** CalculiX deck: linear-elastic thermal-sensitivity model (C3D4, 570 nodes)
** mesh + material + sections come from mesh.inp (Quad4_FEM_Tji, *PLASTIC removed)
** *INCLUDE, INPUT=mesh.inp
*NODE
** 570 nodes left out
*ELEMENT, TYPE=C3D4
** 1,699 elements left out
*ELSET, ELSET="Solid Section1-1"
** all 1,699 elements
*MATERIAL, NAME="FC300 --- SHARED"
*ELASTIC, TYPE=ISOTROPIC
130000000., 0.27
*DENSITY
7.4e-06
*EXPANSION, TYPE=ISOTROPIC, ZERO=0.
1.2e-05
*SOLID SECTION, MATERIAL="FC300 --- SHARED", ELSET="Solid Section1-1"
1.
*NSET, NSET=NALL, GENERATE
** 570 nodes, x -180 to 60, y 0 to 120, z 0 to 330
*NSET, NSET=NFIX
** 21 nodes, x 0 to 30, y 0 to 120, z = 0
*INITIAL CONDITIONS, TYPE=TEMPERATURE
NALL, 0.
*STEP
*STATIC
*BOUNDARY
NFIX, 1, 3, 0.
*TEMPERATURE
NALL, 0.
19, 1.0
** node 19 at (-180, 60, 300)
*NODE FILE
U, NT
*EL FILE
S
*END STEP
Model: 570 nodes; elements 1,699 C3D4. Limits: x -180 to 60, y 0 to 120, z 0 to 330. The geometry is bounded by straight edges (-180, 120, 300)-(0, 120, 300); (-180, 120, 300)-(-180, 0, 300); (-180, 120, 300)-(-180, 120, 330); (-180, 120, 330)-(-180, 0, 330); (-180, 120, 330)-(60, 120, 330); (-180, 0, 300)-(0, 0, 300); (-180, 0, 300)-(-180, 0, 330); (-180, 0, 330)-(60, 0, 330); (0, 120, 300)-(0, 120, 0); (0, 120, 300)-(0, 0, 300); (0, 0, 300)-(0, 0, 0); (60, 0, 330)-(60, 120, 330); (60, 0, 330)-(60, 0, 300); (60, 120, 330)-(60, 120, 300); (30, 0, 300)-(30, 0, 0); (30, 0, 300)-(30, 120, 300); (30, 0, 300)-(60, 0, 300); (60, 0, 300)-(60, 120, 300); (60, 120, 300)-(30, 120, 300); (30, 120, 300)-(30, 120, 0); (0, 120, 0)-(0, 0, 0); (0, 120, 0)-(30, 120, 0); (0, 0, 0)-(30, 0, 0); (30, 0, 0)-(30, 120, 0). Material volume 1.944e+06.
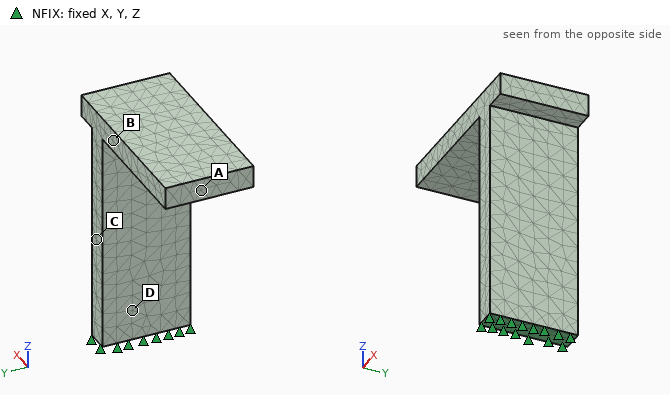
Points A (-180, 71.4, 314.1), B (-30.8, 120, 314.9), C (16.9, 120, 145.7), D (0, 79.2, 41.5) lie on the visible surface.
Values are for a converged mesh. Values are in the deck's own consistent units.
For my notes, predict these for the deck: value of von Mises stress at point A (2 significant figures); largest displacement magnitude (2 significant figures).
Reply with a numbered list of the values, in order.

1. 310
2. 1.7e-04
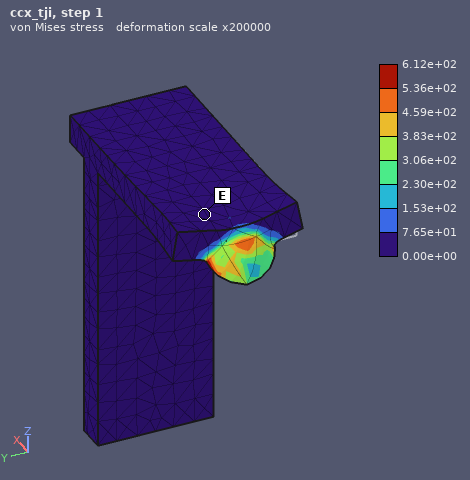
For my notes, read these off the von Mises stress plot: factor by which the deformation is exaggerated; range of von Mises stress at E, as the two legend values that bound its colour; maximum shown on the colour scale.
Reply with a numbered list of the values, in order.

1. 200000
2. 0.00e+00 to 7.65e+01
3. 6.12e+02
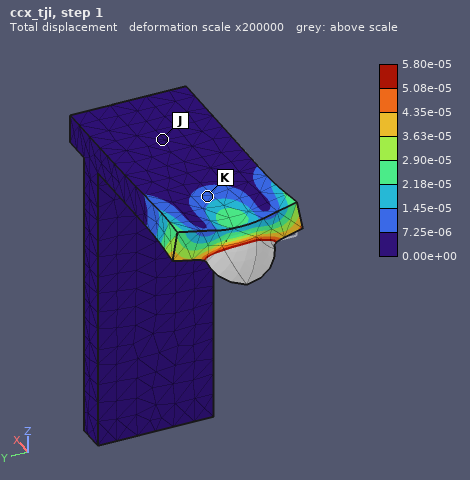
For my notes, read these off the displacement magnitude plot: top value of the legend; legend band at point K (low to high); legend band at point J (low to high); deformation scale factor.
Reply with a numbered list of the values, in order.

1. 5.80e-05
2. 7.25e-06 to 1.45e-05
3. 0.00e+00 to 7.25e-06
4. 200000
